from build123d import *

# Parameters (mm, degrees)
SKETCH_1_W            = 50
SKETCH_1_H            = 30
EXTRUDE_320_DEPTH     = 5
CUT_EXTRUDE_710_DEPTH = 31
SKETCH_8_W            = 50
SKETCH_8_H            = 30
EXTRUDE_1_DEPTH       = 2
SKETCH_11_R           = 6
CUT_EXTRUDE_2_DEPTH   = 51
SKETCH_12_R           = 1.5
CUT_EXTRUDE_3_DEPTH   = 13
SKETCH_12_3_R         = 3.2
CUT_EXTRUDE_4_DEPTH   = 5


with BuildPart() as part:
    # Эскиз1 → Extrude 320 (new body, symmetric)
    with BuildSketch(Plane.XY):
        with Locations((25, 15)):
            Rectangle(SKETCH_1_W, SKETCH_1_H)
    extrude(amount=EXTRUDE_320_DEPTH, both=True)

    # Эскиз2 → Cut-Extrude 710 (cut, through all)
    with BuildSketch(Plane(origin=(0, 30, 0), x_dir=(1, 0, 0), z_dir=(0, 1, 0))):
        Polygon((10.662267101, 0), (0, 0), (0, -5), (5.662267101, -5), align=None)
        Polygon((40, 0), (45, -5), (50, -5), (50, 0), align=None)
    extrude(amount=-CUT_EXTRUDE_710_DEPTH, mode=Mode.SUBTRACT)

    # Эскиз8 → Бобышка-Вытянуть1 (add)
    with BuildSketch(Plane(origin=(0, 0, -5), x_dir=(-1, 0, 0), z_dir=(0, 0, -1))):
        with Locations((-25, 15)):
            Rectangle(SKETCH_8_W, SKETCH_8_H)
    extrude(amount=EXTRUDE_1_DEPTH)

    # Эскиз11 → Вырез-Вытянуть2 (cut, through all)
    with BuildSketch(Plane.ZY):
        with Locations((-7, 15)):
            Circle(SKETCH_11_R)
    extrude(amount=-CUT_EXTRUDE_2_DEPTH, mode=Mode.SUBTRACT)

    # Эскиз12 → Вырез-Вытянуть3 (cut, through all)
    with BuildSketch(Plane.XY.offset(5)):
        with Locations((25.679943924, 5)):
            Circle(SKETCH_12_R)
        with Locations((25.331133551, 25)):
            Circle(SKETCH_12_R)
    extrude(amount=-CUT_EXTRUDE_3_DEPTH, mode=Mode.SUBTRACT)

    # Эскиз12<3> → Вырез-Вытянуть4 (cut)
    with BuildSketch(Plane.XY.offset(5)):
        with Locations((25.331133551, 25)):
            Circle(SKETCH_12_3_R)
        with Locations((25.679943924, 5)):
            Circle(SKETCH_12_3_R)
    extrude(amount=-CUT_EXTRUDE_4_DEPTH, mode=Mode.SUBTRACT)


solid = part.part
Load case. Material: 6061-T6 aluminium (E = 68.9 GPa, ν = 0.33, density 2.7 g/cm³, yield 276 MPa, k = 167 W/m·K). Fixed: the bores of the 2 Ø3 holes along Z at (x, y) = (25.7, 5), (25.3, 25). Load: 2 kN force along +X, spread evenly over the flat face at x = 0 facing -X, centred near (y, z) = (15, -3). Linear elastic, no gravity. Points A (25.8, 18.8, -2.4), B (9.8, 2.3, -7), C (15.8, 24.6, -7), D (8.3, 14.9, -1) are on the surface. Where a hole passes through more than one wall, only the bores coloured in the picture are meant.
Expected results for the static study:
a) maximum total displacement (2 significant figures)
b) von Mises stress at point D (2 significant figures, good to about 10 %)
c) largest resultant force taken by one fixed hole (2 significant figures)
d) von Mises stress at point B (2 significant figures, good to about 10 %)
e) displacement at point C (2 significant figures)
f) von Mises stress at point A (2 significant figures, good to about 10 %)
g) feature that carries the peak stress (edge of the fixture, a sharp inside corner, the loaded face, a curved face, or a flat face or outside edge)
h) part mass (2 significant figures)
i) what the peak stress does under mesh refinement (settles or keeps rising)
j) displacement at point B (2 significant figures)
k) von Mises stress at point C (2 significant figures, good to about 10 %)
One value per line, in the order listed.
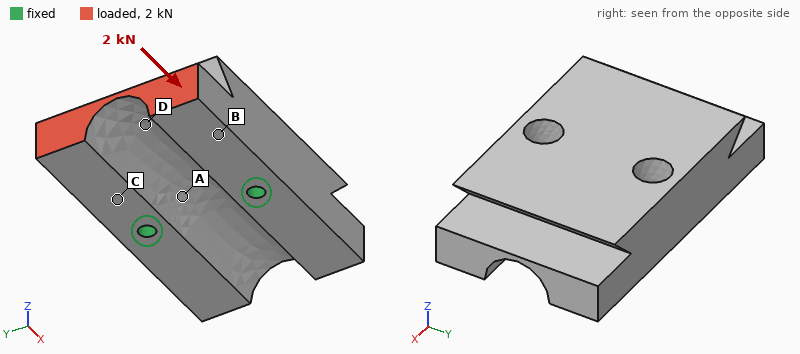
6.8 µm
12 MPa
1.0 kN
14 MPa
2.3 µm
4.2 MPa
edge of the fixture
33 g
keeps rising
4.1 µm
17 MPa
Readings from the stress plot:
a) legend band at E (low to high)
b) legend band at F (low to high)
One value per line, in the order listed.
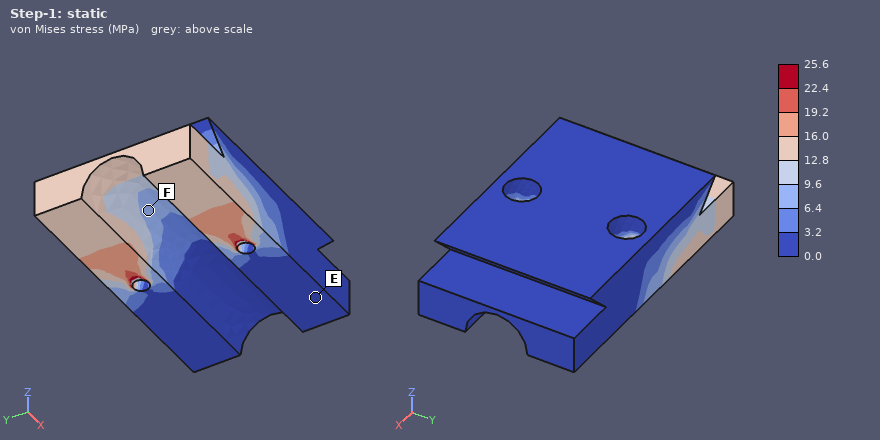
0.0 to 3.2 MPa
6.4 to 9.6 MPa
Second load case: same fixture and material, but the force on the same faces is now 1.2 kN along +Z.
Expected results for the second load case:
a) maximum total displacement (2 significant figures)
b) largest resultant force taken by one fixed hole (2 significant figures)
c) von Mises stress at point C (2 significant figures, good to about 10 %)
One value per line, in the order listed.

95 µm
630 N
55 MPa
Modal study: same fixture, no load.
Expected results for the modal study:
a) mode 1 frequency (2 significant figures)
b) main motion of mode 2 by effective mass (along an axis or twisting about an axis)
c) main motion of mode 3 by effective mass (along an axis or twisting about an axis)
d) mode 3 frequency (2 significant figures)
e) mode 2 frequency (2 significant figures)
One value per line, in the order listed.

8000 Hz
twisting about Z
along Z
14 kHz
13 kHz
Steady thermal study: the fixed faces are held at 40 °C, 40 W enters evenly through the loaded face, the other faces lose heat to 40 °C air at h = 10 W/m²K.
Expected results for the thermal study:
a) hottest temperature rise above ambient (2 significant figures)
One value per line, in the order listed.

33 K
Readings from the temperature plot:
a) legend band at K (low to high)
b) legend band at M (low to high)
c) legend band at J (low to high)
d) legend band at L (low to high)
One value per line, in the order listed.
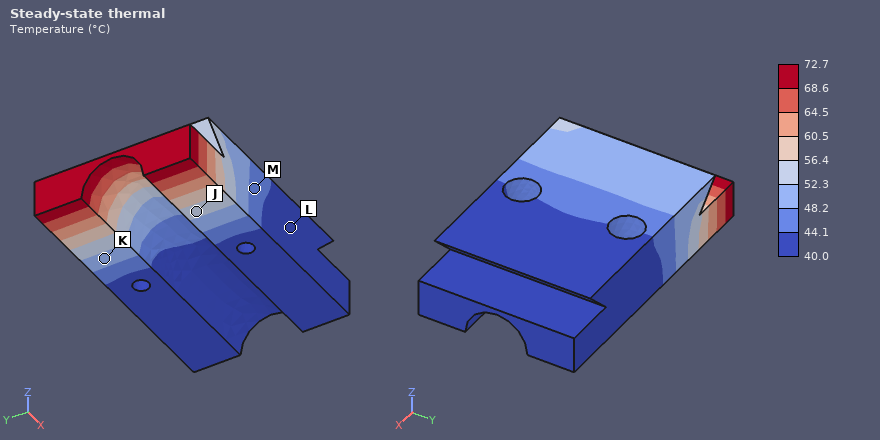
48.2 to 52.3 °C
44.1 to 48.2 °C
52.3 to 56.4 °C
40.0 to 44.1 °C
